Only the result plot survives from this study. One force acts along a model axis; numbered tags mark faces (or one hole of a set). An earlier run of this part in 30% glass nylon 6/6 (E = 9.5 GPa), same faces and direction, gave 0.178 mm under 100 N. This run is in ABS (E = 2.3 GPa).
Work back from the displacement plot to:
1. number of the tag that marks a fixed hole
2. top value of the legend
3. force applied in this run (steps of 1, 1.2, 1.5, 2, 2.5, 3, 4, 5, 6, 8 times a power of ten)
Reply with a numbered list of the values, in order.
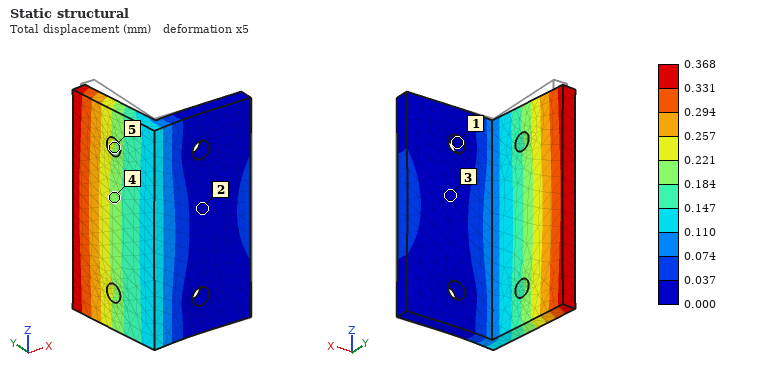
1. 1
2. 0.368 mm
3. 50 N
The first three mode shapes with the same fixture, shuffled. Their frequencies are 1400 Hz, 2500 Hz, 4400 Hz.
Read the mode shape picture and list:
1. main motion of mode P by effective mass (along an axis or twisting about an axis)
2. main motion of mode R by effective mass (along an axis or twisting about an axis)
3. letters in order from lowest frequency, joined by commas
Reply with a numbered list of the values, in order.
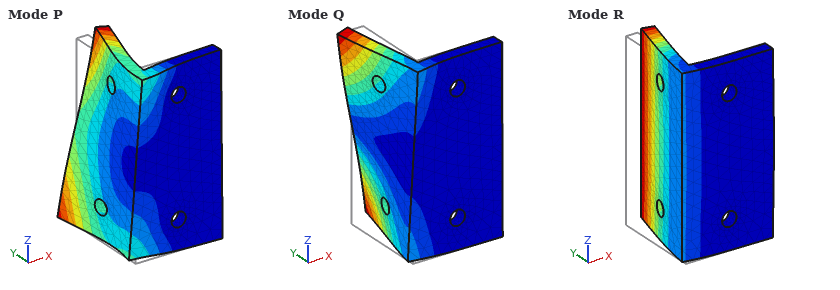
1. along Z
2. along X
3. R, Q, P
